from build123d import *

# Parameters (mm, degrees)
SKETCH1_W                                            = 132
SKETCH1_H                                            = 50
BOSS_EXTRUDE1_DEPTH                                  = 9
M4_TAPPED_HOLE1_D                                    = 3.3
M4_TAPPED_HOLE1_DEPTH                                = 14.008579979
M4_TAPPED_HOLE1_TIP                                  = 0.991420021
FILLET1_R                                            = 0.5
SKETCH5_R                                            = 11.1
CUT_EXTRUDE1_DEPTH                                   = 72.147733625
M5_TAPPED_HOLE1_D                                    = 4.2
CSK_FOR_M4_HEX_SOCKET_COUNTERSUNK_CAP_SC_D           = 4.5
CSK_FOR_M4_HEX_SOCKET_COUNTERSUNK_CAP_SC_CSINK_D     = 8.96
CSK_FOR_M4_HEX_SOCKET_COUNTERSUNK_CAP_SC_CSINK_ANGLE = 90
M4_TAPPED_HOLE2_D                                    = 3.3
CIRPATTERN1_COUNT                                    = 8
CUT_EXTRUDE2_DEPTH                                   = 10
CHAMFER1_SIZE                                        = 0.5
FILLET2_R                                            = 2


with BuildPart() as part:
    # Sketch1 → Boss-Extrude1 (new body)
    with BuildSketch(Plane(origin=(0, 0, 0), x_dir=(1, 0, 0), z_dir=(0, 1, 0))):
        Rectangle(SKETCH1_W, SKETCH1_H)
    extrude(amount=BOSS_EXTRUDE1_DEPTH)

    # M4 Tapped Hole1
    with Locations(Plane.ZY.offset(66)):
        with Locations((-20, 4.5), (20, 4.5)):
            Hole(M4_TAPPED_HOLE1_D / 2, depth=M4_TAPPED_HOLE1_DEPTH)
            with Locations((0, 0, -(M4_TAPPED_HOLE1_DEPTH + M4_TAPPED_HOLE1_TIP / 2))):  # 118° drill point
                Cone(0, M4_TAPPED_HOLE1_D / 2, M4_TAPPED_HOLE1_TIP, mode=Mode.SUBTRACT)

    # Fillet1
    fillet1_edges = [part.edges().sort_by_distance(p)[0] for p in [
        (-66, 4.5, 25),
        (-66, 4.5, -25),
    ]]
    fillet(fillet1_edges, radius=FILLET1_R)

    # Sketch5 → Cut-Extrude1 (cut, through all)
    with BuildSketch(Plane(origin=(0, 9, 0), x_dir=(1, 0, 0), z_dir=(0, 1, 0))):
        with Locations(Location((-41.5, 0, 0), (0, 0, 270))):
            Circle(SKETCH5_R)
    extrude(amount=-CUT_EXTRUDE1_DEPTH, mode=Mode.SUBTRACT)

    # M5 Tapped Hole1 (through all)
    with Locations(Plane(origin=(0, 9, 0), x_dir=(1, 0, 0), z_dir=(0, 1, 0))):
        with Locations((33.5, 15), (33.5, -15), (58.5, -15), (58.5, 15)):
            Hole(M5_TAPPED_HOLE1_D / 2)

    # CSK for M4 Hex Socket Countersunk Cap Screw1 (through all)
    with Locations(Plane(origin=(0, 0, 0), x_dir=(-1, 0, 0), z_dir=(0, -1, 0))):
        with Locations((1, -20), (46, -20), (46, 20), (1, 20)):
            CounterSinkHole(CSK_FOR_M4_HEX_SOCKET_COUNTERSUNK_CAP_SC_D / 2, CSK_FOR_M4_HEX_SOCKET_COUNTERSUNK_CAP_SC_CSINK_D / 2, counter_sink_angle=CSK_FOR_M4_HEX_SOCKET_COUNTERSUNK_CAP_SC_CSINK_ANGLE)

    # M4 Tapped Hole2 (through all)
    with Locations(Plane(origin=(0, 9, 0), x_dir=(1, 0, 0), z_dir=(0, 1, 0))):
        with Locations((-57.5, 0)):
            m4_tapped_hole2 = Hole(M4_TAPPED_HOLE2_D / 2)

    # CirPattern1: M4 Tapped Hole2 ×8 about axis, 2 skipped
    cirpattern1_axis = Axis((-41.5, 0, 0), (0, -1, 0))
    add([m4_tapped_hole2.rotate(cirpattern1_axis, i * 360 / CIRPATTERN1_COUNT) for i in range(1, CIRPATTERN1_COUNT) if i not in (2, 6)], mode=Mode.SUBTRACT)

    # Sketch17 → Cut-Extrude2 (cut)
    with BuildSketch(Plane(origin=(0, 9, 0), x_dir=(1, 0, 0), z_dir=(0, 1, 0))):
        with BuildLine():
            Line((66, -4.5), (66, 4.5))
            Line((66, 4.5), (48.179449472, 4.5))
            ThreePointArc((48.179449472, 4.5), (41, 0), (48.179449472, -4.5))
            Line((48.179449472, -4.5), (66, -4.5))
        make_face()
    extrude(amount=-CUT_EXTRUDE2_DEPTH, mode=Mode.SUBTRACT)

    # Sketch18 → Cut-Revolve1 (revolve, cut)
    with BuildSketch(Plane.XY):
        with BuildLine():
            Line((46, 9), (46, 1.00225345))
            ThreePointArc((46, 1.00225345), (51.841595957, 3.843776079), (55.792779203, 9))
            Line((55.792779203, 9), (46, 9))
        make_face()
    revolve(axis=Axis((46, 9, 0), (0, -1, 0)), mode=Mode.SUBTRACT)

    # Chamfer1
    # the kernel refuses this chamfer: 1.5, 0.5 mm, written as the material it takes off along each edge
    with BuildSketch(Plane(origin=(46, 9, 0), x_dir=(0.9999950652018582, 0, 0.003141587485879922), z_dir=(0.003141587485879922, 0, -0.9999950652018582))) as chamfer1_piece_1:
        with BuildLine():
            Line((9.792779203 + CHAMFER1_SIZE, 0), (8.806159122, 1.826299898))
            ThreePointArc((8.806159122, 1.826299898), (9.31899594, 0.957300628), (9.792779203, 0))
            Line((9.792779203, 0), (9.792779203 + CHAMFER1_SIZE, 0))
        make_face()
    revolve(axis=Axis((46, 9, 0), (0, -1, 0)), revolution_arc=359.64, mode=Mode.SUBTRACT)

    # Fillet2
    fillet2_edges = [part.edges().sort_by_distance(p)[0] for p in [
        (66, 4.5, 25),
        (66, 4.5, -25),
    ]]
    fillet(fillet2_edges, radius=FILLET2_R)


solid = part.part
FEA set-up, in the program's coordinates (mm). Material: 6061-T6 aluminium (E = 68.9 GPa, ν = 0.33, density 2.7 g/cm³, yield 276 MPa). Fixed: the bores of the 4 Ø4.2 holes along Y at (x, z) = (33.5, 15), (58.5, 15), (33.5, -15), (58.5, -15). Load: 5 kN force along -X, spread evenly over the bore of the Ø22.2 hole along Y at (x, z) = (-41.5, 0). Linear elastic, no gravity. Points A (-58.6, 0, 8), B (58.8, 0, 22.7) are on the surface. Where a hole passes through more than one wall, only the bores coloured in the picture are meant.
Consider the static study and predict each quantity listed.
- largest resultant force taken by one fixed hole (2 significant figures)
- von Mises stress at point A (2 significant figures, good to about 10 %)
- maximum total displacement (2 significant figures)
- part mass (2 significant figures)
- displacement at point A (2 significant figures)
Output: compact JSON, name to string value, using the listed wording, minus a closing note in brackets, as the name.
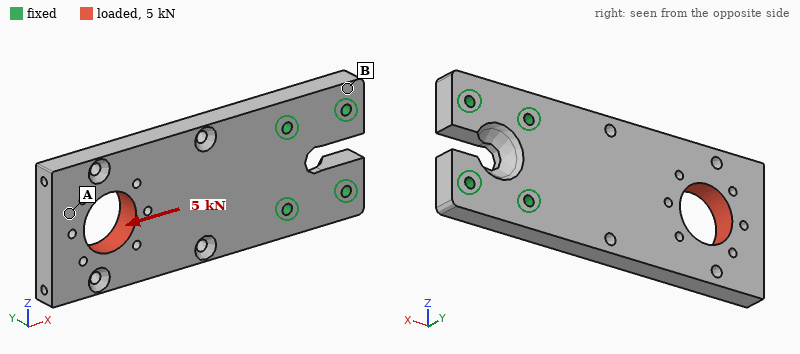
{"largest resultant force taken by one fixed hole": "2.2 kN", "von Mises stress at point A": "8.6 MPa", "maximum total displacement": "22 µm", "part mass": "140 g", "displacement at point A": "20 µm"}
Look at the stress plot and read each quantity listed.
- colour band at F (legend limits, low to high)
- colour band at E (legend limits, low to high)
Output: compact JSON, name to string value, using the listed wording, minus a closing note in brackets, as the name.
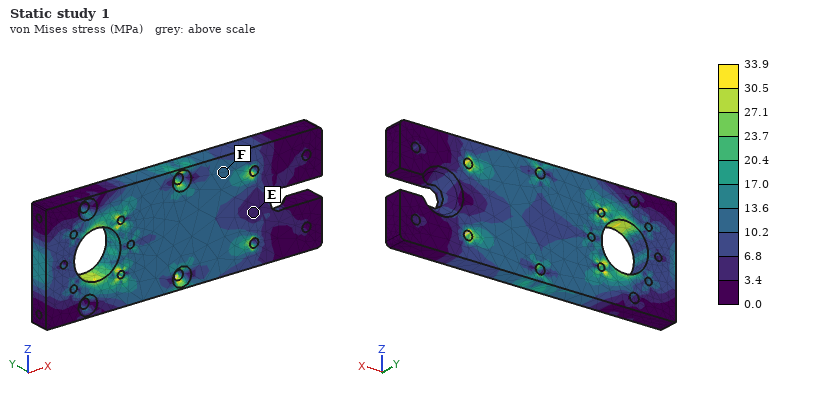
{"colour band at F": "10.2 to 13.6 MPa", "colour band at E": "3.4 to 6.8 MPa"}
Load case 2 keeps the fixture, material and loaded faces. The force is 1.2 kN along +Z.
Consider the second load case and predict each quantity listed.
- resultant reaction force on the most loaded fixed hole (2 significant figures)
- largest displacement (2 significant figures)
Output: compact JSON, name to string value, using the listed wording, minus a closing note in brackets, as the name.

{"resultant reaction force on the most loaded fixed hole": "2.4 kN", "largest displacement": "65 µm"}
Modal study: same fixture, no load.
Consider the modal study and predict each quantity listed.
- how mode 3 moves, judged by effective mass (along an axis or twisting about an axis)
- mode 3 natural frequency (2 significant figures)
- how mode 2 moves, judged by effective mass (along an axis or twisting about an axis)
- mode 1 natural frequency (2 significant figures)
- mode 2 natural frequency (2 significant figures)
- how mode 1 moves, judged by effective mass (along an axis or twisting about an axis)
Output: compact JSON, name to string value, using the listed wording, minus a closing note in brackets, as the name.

{"how mode 3 moves, judged by effective mass": "along Z", "mode 3 natural frequency": "3500 Hz", "how mode 2 moves, judged by effective mass": "twisting about X", "mode 1 natural frequency": "780 Hz", "mode 2 natural frequency": "2800 Hz", "how mode 1 moves, judged by effective mass": "along Y"}
